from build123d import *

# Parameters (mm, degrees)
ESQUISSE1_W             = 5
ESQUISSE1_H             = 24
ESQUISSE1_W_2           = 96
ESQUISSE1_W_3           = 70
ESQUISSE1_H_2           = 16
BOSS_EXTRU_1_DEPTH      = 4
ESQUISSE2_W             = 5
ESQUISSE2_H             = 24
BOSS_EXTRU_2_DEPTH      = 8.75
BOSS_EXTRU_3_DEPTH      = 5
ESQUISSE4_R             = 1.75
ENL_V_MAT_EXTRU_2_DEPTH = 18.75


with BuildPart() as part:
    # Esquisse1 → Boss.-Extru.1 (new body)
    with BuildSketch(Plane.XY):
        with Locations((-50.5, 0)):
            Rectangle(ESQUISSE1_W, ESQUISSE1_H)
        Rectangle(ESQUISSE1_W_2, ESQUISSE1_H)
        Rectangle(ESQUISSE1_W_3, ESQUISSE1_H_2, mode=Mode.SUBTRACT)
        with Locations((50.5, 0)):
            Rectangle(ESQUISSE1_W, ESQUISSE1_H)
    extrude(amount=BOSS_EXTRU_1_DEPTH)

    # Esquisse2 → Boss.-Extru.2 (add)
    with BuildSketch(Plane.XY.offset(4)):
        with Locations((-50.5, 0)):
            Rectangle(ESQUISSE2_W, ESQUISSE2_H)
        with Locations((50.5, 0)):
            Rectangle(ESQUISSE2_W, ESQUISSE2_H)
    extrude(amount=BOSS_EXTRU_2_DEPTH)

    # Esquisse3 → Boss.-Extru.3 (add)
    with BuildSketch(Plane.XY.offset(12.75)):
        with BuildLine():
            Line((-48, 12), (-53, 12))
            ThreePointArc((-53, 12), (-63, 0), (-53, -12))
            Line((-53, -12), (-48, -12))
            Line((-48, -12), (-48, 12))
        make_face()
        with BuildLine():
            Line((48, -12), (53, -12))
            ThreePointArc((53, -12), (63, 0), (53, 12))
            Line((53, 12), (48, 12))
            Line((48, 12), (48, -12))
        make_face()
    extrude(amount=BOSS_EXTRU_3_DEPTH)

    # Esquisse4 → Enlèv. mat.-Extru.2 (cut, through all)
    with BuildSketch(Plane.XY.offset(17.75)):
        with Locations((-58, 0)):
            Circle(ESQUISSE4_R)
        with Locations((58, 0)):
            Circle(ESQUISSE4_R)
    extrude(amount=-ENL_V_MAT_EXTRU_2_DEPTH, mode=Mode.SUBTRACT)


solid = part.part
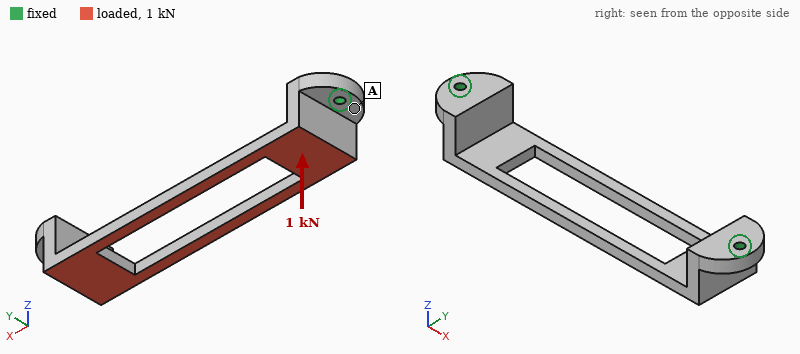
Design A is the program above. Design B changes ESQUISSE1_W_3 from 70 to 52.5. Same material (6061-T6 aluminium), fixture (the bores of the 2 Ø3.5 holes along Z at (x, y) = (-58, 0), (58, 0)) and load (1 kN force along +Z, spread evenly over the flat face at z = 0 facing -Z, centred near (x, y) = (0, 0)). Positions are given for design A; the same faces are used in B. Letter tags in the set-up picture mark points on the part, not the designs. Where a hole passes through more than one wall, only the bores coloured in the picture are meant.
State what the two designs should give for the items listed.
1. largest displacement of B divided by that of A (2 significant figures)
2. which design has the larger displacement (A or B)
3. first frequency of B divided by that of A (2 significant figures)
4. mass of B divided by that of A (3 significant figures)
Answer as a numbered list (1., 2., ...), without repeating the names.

1. 0.88
2. A
3. 1.0
4. 1.10
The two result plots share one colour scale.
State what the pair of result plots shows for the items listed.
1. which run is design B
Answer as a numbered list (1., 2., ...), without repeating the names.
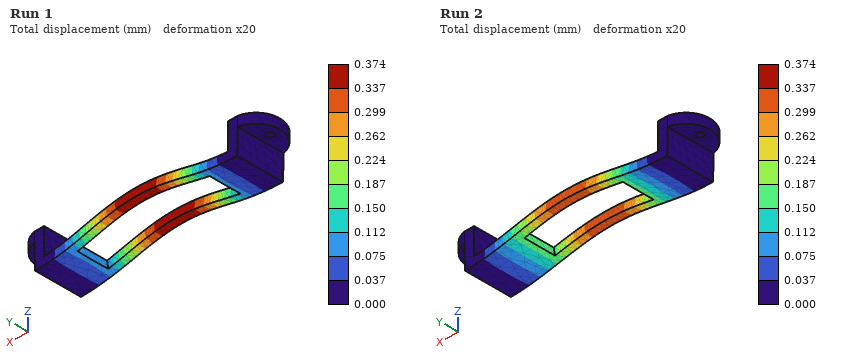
1. Run 2
